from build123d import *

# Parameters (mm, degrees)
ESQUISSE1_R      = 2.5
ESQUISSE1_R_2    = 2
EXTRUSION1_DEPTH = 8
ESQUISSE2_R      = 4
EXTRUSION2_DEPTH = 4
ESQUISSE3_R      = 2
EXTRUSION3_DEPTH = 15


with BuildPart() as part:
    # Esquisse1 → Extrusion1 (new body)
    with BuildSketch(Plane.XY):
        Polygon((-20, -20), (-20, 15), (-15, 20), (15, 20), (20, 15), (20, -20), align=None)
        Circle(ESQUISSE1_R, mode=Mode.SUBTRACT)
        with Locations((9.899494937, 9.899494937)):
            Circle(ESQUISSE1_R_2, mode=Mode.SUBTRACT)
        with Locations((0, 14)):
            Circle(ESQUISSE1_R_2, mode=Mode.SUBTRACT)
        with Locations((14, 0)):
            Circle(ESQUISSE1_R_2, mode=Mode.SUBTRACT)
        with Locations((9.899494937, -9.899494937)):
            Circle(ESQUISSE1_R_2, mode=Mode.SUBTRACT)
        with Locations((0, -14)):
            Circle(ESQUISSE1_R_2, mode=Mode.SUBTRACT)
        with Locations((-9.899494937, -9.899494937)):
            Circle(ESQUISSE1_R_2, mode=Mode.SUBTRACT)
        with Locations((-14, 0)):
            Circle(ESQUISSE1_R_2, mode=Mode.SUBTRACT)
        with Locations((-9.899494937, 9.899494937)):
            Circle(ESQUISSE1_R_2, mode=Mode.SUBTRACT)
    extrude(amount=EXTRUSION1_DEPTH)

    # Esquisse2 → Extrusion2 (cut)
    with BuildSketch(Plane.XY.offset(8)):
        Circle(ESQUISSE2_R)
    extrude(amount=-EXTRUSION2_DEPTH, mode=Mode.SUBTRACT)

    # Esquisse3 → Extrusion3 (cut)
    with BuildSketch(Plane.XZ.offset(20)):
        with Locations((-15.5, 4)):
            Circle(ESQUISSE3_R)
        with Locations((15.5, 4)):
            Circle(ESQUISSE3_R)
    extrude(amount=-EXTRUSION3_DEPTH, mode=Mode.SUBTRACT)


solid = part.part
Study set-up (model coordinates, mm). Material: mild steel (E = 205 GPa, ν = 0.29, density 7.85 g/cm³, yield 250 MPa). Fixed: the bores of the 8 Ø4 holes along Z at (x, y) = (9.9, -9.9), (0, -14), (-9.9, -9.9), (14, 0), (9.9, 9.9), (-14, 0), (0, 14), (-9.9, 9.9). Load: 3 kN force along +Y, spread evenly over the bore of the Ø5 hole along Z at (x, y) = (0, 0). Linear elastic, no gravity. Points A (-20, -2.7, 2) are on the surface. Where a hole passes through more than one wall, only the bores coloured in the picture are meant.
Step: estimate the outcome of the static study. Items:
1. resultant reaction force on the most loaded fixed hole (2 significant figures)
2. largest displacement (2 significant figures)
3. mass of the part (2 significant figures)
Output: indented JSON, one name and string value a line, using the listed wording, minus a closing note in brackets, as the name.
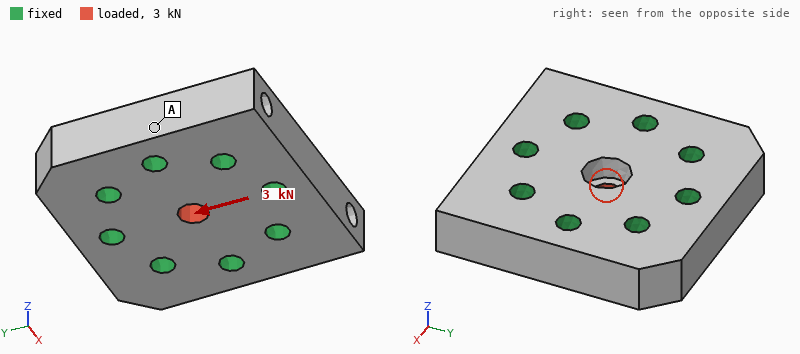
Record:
{
  "resultant reaction force on the most loaded fixed hole": "670 N",
  "largest displacement": "1.4 µm",
  "mass of the part": "87 g"
}
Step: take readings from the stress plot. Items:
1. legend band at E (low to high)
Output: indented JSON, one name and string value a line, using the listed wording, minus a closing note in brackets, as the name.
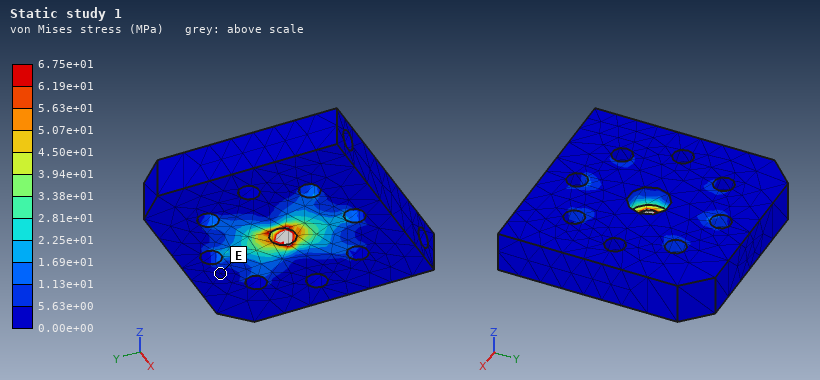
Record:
{
  "legend band at E": "0.00e+00 to 5.63e+00 MPa"
}
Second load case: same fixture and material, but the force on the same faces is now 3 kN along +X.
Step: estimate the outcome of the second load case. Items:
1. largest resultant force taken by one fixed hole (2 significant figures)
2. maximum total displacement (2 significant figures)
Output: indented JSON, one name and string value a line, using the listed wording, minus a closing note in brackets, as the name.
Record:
{
  "largest resultant force taken by one fixed hole": "680 N",
  "maximum total displacement": "1.4 µm"
}
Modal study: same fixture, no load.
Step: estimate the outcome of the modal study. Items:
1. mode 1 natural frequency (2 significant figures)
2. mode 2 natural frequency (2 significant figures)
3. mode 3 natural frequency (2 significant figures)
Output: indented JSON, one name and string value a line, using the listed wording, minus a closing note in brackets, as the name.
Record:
{
  "mode 1 natural frequency": "42 kHz",
  "mode 2 natural frequency": "42 kHz",
  "mode 3 natural frequency": "52 kHz"
}
